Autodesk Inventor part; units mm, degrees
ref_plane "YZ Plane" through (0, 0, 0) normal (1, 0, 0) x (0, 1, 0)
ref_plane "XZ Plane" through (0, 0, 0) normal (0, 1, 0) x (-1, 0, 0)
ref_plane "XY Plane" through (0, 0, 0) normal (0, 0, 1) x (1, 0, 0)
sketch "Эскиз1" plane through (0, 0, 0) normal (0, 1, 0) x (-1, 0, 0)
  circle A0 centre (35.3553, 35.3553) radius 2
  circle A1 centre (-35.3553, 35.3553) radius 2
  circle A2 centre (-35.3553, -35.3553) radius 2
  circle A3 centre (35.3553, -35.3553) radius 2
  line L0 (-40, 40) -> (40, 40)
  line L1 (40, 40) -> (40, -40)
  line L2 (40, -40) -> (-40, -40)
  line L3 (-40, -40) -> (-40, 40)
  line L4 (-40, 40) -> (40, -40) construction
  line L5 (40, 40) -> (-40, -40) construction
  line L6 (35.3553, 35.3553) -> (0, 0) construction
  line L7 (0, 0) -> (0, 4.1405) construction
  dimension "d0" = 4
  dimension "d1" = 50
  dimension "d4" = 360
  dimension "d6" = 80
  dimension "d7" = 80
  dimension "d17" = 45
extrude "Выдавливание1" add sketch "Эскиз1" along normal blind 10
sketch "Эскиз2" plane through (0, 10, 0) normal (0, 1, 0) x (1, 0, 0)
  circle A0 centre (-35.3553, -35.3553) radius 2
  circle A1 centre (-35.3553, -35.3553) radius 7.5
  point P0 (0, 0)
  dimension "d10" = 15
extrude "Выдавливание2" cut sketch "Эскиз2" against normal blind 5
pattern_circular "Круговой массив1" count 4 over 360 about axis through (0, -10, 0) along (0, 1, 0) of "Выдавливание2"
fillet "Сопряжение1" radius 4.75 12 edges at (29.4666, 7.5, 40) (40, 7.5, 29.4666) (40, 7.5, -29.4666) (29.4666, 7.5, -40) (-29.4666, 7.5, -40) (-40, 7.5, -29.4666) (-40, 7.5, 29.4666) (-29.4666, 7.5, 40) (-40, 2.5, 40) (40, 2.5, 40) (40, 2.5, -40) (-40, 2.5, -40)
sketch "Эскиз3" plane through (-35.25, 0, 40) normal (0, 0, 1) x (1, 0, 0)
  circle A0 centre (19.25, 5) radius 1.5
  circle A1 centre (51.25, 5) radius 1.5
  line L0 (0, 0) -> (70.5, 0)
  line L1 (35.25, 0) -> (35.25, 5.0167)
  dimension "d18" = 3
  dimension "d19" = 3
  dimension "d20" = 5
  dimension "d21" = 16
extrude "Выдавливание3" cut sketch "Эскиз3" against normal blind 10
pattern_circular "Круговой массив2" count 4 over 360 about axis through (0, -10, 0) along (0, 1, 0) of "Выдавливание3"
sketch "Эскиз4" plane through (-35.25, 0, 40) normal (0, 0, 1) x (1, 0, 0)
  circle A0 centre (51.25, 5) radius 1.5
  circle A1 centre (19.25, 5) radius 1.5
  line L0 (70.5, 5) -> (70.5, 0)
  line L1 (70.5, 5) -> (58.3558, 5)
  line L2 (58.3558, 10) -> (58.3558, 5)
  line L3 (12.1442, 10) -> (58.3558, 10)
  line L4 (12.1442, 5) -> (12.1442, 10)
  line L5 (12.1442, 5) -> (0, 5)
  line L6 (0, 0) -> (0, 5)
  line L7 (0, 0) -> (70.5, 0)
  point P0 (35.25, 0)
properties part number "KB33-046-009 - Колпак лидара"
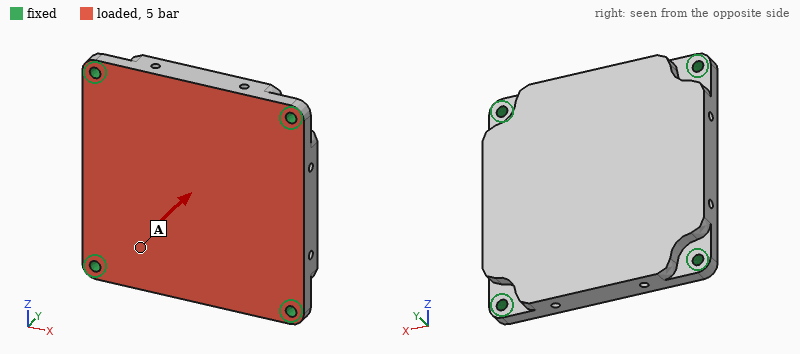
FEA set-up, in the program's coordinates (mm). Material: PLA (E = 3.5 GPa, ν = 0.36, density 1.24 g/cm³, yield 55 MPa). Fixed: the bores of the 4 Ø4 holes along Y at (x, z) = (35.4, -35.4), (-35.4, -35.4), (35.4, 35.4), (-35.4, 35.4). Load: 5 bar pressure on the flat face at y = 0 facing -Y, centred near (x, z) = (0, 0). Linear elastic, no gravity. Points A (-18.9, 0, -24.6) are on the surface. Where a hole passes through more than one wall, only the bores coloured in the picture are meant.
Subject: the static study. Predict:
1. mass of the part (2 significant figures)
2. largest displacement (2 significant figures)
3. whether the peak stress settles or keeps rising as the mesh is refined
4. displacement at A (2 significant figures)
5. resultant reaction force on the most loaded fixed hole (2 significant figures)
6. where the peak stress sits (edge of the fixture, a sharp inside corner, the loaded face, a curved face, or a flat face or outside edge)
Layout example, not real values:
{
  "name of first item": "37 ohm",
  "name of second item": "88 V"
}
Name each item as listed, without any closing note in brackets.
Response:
{
  "mass of the part": "75 g",
  "largest displacement": "0.58 mm",
  "whether the peak stress settles or keeps rising as the mesh is refined": "keeps rising",
  "displacement at A": "0.37 mm",
  "resultant reaction force on the most loaded fixed hole": "1.1 kN",
  "where the peak stress sits": "edge of the fixture"
}
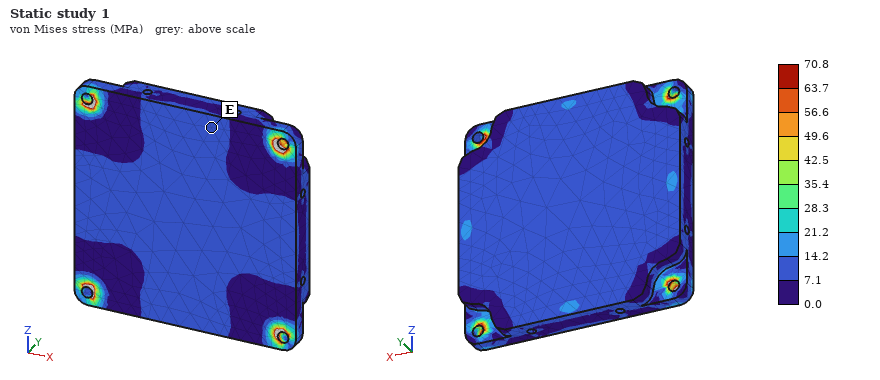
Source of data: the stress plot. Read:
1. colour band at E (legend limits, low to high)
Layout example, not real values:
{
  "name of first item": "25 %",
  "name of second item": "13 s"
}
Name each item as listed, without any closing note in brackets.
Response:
{
  "colour band at E": "7.1 to 14.2 MPa"
}
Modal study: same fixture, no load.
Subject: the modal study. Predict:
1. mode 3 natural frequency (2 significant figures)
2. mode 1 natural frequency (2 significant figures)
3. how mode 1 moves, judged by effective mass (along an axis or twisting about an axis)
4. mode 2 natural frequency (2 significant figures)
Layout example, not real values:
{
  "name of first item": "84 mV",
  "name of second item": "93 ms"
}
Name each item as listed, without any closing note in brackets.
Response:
{
  "mode 3 natural frequency": "2600 Hz",
  "mode 1 natural frequency": "1500 Hz",
  "how mode 1 moves, judged by effective mass": "along Y",
  "mode 2 natural frequency": "2600 Hz"
}
